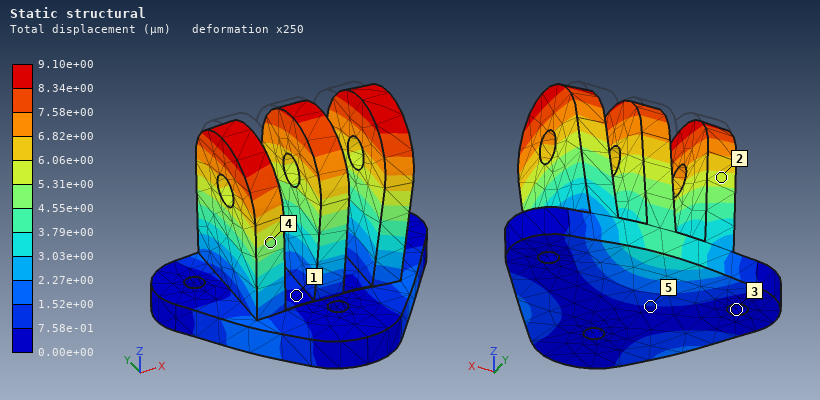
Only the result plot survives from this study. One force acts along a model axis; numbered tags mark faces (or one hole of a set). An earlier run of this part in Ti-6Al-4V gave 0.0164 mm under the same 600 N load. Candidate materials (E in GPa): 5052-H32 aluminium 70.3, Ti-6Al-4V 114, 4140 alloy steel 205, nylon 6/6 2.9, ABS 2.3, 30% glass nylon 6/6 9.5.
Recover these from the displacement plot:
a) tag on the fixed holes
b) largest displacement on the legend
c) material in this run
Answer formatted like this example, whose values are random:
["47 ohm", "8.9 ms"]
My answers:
["3", "9.10e+00 µm", "4140 alloy steel"]
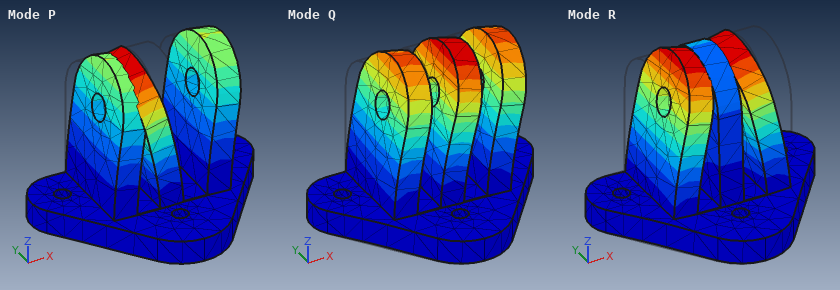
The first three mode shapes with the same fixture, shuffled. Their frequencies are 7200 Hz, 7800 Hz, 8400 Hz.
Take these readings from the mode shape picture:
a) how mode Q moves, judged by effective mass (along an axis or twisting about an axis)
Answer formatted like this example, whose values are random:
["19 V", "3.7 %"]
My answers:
["along X"]
